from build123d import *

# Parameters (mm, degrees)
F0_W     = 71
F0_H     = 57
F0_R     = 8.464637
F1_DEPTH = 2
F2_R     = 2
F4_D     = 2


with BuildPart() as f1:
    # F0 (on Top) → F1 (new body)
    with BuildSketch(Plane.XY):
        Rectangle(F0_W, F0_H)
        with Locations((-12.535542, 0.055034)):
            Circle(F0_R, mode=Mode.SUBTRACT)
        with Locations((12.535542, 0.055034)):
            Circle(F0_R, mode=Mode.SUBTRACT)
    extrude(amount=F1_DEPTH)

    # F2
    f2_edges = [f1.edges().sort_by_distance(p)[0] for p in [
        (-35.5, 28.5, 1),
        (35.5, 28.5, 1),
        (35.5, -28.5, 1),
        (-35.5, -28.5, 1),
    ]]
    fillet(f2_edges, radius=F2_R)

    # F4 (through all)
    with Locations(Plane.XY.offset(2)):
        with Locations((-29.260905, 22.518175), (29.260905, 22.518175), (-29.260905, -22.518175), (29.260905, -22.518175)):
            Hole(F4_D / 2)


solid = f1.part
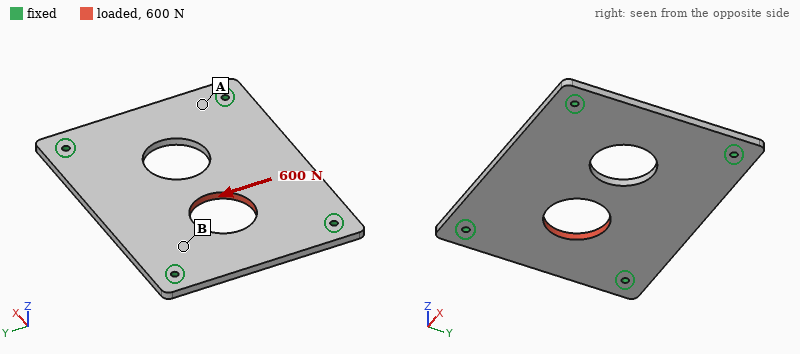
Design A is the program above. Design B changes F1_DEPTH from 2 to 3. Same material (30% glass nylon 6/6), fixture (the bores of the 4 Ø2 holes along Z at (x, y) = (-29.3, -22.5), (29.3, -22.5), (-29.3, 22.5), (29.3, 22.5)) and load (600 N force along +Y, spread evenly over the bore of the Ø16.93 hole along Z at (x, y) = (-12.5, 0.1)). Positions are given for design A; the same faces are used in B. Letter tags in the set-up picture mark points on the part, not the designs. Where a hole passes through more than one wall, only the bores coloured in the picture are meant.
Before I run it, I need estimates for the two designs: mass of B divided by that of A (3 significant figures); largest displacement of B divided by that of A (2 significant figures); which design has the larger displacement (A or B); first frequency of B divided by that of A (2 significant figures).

1.50
0.67
A
1.4
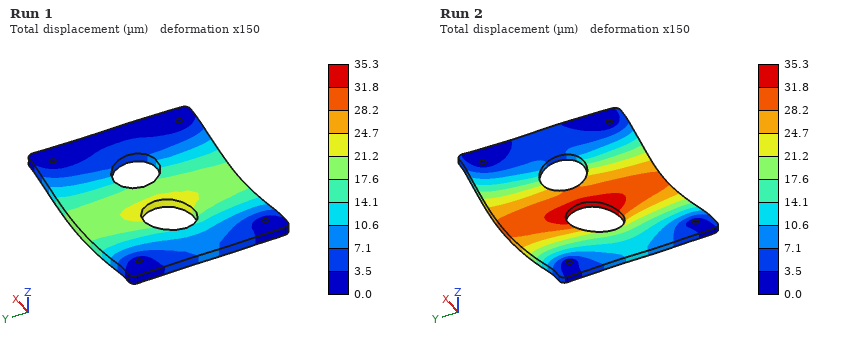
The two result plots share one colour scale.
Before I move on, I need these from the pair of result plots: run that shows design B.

Run 1
